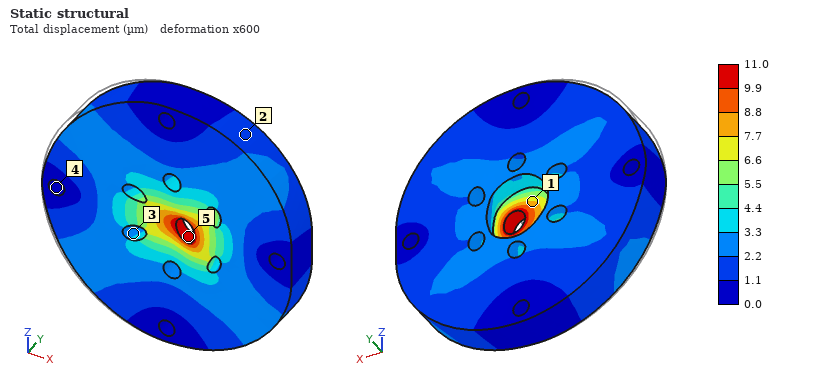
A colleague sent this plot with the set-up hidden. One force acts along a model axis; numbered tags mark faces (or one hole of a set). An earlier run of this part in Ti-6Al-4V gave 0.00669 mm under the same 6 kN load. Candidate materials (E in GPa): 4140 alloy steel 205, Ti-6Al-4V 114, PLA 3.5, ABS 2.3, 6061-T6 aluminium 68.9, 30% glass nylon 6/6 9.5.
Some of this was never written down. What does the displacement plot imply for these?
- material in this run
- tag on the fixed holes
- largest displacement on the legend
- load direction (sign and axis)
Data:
6061-T6 aluminium
4
11.0 µm
+X
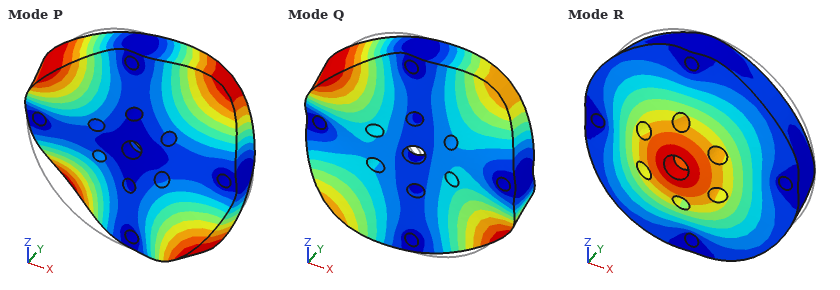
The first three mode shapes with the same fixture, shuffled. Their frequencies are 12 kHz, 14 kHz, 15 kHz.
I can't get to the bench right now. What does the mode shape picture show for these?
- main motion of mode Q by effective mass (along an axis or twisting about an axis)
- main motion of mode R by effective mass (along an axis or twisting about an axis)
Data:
twisting about Z
along Y
